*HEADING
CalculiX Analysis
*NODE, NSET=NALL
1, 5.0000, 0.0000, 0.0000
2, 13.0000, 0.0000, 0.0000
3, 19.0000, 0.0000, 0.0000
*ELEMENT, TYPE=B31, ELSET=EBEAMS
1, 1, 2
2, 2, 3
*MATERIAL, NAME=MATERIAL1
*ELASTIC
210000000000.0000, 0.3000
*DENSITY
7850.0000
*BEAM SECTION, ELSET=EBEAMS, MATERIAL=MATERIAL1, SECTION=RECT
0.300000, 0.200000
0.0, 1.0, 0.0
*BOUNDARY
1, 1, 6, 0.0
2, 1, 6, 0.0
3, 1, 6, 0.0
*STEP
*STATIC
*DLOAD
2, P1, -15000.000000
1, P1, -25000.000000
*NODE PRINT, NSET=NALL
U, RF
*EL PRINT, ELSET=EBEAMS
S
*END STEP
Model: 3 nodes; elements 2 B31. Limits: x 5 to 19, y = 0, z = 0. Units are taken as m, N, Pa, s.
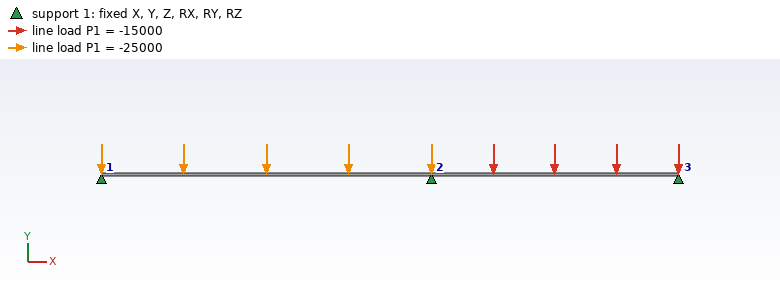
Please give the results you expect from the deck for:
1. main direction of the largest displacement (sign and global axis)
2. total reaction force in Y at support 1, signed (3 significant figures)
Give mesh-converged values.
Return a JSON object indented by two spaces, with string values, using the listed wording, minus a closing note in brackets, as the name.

{
  "main direction of the largest displacement": "-Y",
  "total reaction force in Y at support 1, signed": "2.90e+05 N"
}
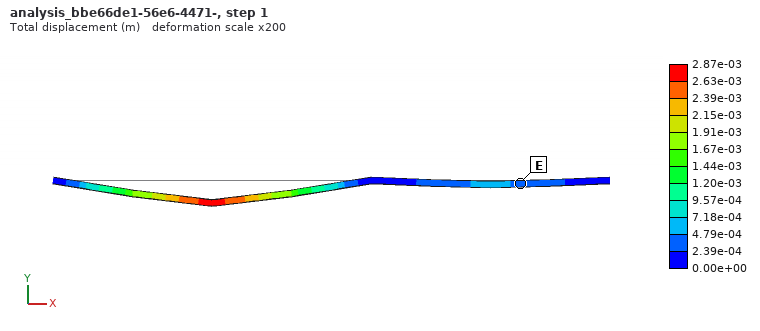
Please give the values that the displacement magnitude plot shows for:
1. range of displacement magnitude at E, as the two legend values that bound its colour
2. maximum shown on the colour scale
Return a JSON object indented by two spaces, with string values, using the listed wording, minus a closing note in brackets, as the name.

{
  "range of displacement magnitude at E, as the two legend values that bound its colour": "2.39e-04 to 4.79e-04 m",
  "maximum shown on the colour scale": "2.87e-03 m"
}
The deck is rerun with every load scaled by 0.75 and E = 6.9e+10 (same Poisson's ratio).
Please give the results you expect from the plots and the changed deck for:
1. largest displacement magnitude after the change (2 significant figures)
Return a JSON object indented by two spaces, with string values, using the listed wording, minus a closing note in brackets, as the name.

{
  "largest displacement magnitude after the change": "0.0066 m"
}
